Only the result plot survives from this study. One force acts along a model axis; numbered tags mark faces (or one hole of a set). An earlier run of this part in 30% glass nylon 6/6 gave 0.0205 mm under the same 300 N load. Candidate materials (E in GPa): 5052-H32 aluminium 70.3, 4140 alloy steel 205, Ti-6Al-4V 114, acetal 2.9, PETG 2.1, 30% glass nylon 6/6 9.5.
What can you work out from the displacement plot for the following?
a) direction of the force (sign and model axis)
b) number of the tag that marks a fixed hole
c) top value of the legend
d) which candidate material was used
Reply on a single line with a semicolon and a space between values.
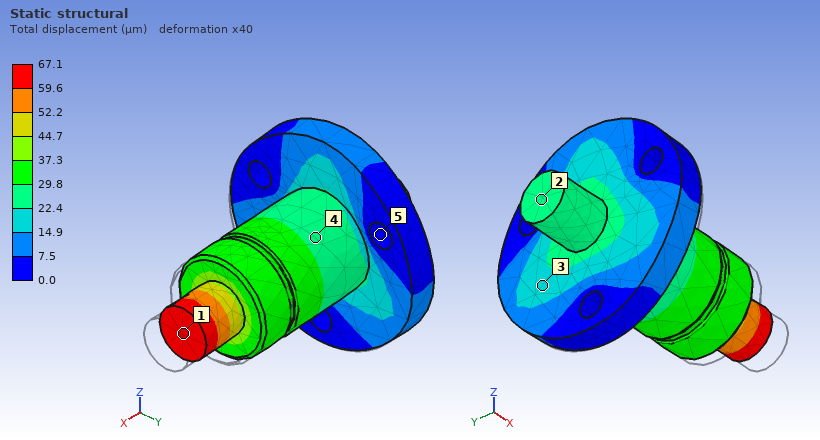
-X; 5; 67.1 µm; acetal
